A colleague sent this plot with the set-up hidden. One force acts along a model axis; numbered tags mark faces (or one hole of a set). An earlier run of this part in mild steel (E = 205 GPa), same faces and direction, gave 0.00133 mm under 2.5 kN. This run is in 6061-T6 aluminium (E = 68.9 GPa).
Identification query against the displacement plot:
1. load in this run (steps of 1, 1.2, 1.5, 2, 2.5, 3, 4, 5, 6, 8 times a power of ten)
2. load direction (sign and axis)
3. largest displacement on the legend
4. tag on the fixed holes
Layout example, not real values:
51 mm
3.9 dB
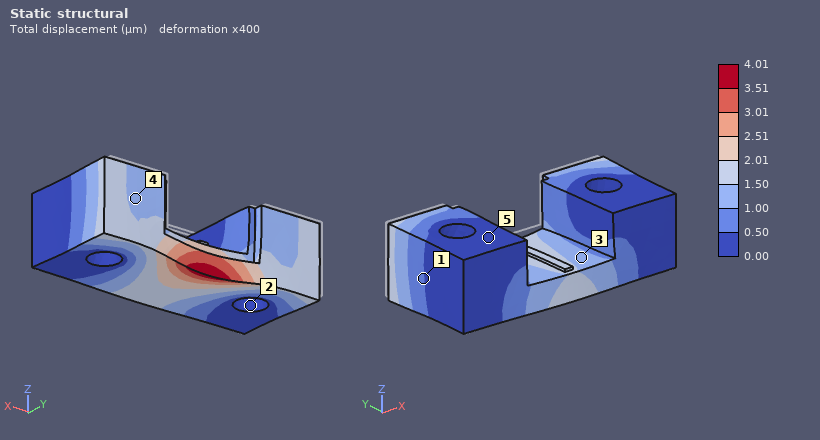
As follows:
2.5 kN
-Y
4.01 µm
2
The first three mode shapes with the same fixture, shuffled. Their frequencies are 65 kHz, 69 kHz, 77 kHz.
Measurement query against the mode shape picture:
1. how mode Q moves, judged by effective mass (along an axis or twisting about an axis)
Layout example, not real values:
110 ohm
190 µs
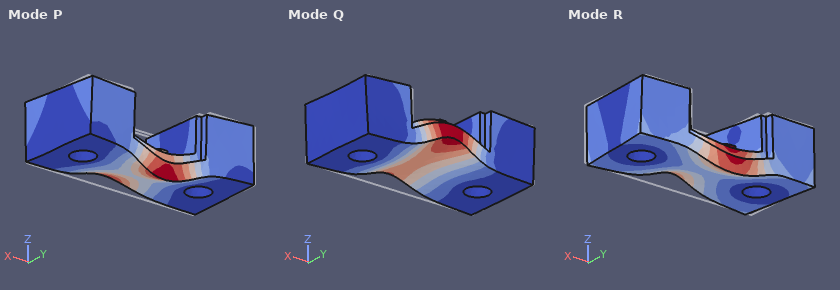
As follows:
along Z
